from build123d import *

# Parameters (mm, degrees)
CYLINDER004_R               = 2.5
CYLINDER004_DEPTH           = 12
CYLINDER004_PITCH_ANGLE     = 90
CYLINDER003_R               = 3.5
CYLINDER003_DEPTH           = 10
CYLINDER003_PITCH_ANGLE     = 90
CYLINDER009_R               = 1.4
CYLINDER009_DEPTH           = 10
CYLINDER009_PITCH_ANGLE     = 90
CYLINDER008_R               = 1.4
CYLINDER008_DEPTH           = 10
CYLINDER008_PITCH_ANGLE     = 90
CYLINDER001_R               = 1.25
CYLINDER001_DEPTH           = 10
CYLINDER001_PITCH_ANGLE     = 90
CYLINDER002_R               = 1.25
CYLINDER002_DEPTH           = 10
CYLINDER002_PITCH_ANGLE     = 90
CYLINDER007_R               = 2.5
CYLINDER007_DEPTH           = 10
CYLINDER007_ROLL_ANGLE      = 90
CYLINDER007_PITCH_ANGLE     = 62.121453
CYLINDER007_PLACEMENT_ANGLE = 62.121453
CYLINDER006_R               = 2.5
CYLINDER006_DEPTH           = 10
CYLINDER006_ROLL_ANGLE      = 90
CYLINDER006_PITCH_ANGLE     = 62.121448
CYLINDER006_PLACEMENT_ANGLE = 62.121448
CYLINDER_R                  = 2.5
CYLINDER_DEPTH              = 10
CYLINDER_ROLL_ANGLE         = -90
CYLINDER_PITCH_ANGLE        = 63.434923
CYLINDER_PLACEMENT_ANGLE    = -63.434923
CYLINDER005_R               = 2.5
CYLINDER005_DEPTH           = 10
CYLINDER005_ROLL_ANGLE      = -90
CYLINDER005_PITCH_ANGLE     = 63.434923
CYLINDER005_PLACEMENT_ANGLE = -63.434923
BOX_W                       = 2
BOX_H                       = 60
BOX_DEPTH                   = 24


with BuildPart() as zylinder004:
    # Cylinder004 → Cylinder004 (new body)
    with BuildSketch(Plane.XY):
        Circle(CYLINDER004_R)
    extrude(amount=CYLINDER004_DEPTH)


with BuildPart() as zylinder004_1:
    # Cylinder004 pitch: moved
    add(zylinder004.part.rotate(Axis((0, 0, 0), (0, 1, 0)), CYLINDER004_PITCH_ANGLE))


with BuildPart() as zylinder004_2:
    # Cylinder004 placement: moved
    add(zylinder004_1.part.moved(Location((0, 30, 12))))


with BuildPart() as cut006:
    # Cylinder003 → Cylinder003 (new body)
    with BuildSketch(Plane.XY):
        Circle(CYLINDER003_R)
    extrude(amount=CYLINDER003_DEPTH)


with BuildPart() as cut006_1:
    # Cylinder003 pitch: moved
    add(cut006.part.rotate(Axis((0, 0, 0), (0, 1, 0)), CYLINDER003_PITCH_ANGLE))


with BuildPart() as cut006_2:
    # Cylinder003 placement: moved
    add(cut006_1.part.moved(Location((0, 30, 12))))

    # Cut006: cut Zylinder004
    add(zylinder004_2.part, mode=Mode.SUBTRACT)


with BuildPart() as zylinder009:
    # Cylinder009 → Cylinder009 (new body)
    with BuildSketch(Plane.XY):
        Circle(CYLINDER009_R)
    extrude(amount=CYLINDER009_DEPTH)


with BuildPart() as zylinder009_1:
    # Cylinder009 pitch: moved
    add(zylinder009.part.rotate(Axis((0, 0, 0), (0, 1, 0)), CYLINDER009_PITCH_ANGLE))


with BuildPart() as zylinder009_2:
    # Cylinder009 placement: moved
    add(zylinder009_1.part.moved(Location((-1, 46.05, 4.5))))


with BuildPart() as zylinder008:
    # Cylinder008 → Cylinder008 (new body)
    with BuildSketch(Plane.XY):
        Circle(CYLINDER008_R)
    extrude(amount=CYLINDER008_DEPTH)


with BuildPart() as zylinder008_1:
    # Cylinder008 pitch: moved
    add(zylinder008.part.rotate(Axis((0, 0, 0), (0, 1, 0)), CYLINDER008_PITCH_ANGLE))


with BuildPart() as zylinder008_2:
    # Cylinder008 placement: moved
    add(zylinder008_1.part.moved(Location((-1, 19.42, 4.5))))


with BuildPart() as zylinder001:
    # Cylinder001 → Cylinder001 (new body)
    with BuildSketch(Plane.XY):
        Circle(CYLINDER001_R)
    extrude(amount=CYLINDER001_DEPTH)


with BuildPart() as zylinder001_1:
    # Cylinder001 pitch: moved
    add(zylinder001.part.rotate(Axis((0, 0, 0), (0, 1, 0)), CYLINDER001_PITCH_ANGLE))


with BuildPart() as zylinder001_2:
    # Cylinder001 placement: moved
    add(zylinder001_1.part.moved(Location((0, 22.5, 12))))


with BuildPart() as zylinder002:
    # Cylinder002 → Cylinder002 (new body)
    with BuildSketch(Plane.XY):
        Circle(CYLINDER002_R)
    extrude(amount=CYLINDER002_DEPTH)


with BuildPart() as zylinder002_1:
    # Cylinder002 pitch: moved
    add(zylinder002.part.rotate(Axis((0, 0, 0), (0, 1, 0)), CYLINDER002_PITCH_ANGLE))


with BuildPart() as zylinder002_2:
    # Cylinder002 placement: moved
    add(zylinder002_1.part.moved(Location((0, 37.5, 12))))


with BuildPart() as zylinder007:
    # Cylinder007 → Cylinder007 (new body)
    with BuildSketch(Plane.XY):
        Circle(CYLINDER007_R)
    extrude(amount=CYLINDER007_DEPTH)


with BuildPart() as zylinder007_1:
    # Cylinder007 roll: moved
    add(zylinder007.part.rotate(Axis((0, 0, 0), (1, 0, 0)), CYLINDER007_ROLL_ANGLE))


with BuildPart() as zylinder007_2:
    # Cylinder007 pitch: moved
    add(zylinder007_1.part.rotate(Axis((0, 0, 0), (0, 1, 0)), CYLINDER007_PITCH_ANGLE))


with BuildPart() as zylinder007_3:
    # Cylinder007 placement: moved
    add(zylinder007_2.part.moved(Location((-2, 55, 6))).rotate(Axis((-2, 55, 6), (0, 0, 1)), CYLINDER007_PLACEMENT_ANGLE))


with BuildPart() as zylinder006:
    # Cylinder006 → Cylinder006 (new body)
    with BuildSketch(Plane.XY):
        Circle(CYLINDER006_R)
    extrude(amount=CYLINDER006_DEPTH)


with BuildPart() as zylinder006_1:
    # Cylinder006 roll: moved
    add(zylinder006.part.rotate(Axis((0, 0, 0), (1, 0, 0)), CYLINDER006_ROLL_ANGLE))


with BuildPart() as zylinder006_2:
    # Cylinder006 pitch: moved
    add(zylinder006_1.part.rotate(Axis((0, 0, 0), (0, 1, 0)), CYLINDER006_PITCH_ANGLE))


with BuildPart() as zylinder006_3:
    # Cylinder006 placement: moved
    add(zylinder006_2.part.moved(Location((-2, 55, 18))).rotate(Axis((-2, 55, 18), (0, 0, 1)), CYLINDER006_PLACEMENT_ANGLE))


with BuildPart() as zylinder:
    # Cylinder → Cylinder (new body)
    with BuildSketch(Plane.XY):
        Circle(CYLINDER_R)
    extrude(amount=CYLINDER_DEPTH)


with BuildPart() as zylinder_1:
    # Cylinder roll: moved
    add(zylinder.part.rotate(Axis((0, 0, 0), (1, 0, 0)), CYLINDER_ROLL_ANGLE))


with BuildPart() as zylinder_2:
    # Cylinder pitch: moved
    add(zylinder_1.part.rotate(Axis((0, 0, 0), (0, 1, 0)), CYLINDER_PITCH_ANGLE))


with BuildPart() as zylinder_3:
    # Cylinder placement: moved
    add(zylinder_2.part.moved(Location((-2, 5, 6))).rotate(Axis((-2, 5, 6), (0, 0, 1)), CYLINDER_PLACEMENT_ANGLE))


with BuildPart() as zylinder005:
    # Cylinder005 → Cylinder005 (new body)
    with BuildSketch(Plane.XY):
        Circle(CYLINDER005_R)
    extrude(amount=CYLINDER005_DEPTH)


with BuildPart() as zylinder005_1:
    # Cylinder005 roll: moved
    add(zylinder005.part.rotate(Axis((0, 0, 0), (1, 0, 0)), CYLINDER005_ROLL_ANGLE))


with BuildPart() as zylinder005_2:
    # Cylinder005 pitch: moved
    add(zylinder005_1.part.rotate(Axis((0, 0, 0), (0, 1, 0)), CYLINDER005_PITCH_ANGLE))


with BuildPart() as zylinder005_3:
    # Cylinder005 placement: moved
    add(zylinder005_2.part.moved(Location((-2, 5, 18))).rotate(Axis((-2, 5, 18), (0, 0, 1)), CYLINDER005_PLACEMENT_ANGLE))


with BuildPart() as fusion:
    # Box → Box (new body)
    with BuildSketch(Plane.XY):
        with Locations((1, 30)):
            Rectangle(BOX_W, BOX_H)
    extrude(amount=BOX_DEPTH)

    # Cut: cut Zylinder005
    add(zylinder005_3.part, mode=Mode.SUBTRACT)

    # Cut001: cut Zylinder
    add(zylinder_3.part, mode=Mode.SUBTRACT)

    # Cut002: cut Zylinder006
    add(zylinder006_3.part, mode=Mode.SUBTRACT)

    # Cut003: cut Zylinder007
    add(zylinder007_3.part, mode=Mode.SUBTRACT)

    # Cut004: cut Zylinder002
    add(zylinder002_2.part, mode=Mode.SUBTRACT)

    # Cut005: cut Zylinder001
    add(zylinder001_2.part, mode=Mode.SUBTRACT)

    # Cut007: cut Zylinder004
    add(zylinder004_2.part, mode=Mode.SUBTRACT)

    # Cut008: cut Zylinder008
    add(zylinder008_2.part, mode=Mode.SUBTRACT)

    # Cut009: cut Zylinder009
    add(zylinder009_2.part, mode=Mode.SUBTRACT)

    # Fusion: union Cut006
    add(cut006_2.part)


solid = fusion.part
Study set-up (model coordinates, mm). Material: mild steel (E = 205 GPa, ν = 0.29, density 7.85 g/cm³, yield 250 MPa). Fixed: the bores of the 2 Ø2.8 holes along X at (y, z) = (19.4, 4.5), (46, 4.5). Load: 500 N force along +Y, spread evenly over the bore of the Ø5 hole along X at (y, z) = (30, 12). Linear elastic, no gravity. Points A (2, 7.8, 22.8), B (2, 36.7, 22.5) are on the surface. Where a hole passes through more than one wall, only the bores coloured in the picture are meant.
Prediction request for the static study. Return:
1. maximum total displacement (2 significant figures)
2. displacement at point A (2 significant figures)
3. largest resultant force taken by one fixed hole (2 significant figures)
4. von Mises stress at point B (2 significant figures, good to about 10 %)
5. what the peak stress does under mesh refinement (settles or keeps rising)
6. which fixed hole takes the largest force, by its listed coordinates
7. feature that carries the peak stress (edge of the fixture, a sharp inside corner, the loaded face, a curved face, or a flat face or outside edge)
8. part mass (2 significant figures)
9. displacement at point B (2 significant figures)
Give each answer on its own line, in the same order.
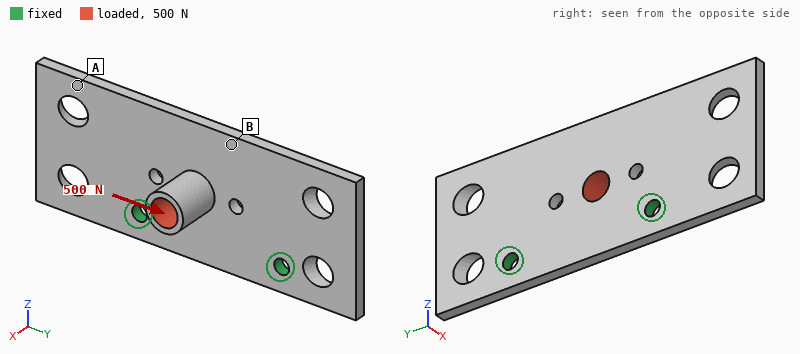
22 µm
8.8 µm
310 N
27 MPa
keeps rising
(19.4, 4.5)
edge of the fixture
22 g
9.5 µm
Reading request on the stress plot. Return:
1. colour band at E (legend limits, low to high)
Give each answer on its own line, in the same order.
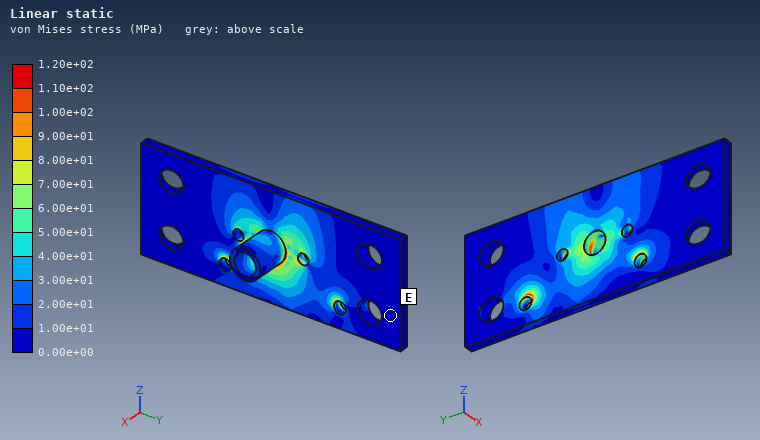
0.00e+00 to 1.00e+01 MPa
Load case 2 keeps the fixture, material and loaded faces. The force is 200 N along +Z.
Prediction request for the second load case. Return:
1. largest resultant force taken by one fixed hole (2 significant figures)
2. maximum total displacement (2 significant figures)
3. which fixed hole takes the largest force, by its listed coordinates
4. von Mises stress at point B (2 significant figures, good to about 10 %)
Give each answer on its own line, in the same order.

130 N
23 µm
(19.4, 4.5)
7.1 MPa
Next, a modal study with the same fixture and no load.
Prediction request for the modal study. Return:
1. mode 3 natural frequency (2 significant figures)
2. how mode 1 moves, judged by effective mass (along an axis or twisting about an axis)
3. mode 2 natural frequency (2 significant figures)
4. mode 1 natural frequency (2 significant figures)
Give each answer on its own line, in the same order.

5000 Hz
along X
3800 Hz
3200 Hz
